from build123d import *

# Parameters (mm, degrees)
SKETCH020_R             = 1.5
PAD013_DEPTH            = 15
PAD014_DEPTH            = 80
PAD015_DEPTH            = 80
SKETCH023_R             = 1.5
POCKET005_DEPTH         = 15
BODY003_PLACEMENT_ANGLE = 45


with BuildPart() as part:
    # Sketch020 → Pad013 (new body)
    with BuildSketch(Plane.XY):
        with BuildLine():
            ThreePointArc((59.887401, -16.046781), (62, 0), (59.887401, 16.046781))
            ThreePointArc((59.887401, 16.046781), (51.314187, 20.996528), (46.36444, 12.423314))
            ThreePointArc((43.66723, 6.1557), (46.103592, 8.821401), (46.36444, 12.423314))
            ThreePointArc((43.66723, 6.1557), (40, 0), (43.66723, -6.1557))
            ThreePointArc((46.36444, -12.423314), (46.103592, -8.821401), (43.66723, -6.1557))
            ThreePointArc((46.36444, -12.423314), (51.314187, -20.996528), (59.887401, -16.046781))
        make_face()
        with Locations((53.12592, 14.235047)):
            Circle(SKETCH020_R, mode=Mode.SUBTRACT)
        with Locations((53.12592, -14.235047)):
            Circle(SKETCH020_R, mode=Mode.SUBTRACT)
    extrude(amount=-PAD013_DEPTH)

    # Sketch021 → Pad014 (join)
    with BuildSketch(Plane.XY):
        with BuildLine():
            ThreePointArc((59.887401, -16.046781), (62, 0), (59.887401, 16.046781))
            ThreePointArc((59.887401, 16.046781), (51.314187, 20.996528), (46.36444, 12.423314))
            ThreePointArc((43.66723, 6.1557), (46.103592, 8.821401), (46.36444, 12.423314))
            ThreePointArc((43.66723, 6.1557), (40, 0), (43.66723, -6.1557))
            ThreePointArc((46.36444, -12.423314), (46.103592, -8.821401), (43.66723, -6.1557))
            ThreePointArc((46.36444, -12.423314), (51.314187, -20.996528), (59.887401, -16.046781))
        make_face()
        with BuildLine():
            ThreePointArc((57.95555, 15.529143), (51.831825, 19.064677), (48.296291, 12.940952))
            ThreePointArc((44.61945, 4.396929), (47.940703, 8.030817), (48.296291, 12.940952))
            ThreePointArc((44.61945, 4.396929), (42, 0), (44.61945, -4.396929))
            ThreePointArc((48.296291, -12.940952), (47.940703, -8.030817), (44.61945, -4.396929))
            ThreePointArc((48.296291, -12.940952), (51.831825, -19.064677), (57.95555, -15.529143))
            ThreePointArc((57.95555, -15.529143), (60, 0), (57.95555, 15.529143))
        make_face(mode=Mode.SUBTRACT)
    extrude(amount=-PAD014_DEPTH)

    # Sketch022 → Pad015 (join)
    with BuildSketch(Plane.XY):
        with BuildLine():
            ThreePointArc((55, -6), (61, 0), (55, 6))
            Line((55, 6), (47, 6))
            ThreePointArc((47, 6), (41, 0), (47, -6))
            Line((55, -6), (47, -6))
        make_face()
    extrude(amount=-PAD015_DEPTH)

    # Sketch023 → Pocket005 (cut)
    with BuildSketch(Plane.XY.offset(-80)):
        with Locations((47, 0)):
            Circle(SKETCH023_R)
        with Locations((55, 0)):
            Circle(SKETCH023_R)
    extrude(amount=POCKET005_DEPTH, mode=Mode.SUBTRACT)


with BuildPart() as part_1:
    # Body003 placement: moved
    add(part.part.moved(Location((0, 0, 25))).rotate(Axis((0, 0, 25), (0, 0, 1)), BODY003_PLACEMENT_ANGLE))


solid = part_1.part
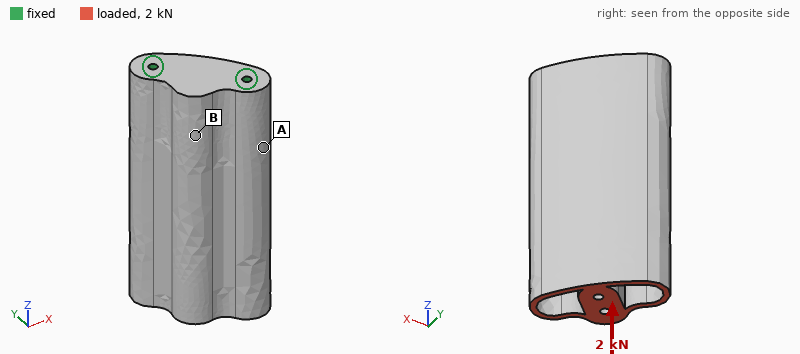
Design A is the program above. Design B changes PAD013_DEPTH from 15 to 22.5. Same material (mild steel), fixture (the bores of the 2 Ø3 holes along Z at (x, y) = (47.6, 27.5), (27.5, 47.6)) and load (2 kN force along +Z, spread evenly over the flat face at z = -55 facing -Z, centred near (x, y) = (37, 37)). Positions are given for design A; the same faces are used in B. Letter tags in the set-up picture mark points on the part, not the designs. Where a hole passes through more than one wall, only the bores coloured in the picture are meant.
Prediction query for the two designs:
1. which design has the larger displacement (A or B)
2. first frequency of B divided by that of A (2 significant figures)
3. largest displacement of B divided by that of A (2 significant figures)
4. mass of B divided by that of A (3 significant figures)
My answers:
A
1.3
0.75
1.05
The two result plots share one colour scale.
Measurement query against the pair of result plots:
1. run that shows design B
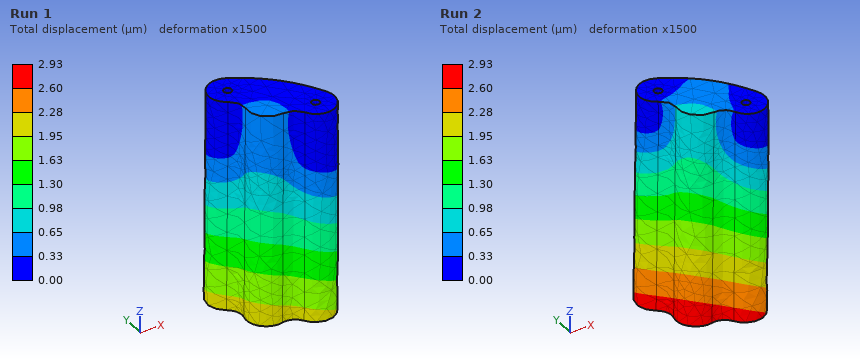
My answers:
Run 1
